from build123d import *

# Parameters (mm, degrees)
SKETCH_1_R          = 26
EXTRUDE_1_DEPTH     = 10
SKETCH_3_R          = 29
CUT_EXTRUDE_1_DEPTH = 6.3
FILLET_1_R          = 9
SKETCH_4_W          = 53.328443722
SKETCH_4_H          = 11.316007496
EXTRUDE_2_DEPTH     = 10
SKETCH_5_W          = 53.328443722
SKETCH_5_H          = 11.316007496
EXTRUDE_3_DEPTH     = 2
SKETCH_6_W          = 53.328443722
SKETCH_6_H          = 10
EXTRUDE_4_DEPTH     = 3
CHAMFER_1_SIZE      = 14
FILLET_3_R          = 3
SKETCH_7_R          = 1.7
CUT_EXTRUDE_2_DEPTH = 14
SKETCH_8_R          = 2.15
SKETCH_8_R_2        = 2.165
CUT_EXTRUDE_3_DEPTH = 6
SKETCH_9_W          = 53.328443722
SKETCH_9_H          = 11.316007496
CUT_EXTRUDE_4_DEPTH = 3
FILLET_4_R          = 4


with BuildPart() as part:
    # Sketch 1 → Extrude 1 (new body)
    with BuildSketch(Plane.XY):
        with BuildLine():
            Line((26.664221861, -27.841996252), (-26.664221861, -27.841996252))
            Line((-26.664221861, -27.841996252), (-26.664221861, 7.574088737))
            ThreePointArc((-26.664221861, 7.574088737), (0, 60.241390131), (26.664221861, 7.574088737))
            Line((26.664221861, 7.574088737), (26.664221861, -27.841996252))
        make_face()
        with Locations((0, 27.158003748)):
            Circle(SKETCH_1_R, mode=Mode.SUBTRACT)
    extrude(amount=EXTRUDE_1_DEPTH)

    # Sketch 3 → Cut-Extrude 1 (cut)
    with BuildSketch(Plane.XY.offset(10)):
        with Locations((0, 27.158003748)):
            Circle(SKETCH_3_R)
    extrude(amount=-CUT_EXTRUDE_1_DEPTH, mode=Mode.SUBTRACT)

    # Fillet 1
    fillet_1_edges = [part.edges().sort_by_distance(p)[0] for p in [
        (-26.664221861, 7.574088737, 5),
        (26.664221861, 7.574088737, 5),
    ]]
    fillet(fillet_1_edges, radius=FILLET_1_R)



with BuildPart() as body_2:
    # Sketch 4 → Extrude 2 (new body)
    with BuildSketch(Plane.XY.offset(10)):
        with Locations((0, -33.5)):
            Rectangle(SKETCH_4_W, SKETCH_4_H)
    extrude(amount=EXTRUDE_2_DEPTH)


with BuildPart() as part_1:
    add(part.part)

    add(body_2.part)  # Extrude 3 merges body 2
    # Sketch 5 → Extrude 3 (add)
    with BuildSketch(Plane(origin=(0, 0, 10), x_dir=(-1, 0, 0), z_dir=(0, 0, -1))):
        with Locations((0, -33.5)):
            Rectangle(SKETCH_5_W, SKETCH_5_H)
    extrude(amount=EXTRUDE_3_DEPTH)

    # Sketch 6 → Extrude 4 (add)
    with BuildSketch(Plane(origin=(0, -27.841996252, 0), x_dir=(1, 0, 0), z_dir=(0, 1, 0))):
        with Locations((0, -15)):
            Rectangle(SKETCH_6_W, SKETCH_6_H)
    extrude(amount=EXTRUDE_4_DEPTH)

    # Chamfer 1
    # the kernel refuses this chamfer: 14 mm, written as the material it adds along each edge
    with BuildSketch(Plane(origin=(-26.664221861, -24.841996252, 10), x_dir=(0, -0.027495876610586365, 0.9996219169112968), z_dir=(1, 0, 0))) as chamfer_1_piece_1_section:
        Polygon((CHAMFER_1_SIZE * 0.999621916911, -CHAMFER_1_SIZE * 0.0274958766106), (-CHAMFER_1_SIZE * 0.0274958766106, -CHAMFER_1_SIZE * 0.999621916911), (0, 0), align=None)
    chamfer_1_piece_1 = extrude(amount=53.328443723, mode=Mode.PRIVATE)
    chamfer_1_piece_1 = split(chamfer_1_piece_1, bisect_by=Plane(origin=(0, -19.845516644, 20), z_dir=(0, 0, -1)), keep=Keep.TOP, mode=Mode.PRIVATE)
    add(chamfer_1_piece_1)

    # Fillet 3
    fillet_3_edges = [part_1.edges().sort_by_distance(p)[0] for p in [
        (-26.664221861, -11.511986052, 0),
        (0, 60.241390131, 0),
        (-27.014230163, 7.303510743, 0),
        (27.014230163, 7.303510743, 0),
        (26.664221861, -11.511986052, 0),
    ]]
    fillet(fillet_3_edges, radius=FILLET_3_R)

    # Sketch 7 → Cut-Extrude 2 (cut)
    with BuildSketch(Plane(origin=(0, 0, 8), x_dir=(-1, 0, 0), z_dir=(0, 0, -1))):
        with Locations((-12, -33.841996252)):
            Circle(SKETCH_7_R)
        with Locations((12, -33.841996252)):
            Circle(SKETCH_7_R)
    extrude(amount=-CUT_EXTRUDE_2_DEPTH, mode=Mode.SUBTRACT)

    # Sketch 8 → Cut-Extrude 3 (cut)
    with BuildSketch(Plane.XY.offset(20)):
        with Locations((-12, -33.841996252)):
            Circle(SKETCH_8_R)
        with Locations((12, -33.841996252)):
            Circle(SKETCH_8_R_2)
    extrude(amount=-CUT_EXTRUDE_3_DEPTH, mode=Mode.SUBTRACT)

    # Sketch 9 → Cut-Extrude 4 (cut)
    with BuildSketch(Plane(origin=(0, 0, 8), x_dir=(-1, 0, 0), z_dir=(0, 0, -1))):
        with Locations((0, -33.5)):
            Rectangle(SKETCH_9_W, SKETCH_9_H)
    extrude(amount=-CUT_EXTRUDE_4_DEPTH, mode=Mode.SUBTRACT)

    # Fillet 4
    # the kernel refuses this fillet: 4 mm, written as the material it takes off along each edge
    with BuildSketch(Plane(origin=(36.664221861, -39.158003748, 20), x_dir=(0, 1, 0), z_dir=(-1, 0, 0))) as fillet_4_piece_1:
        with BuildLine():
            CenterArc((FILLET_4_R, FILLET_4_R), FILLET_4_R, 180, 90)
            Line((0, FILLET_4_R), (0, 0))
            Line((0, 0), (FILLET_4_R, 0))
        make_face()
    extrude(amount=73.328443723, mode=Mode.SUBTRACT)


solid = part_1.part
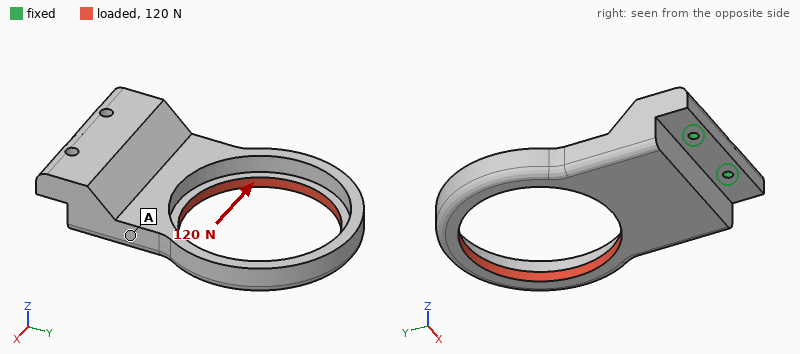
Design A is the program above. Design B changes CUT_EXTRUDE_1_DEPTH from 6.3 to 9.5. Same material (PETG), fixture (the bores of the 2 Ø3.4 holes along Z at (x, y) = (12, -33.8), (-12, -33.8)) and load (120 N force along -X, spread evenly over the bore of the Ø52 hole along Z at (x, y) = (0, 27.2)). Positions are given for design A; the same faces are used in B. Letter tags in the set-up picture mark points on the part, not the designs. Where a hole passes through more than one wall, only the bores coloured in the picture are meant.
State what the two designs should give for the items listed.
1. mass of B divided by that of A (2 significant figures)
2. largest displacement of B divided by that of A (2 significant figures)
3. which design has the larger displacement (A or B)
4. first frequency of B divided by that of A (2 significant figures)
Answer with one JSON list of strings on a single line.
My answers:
["0.95", "1.7", "B", "1.1"]
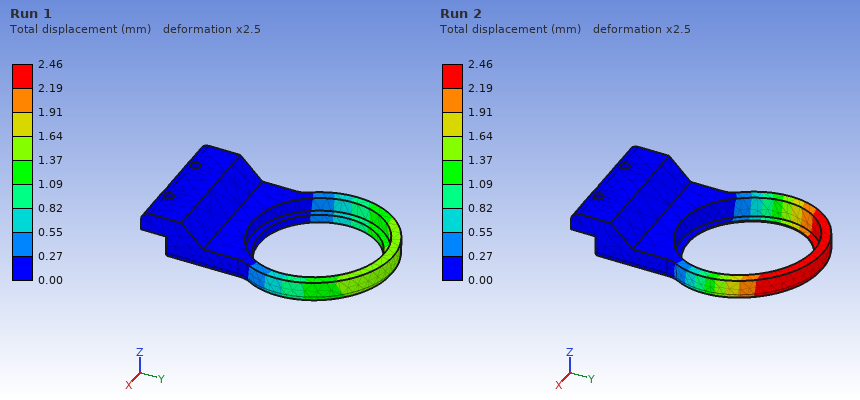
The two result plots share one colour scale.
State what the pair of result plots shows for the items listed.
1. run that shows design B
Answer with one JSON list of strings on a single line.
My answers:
["Run 2"]
